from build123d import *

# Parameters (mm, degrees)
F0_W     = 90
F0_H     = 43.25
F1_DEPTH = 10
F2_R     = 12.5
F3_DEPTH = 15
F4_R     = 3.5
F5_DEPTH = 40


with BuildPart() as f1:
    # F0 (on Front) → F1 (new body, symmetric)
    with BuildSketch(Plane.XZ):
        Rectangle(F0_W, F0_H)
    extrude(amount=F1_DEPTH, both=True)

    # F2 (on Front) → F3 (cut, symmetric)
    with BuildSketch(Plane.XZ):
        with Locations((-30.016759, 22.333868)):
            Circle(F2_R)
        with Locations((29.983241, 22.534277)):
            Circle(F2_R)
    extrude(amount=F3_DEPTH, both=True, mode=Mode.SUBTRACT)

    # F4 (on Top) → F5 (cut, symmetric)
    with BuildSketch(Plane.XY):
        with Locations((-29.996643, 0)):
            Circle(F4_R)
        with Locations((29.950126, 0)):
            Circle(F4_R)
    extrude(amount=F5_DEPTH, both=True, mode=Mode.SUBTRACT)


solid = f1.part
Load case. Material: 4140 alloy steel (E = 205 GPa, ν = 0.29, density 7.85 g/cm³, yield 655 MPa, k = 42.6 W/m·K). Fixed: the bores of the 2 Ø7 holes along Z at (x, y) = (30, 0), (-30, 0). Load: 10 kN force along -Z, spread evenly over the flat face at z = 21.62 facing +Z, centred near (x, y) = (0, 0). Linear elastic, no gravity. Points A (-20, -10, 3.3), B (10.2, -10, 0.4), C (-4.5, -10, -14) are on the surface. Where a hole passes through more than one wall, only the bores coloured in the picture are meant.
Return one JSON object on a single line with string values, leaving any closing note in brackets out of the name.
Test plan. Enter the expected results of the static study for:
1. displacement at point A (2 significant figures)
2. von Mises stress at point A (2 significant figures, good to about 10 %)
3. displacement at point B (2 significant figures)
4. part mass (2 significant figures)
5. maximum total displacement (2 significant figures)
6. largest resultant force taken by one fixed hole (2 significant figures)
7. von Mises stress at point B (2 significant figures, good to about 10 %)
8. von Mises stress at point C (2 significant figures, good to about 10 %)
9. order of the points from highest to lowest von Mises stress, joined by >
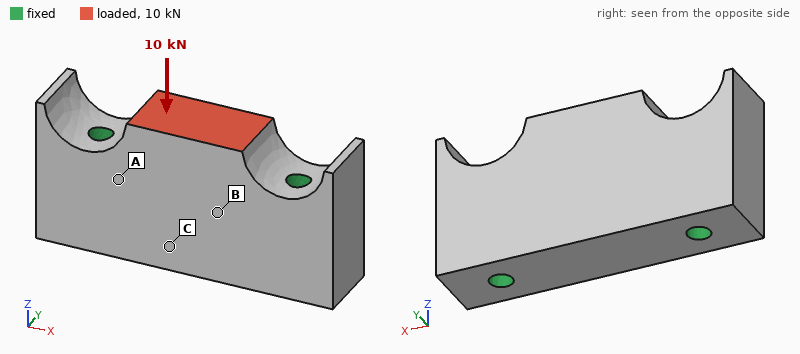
{"displacement at point A": "1.2 µm", "von Mises stress at point A": "15 MPa", "displacement at point B": "1.9 µm", "part mass": "520 g", "maximum total displacement": "3.3 µm", "largest resultant force taken by one fixed hole": "5.3 kN", "von Mises stress at point B": "10 MPa", "von Mises stress at point C": "4.2 MPa", "order of the points from highest to lowest von Mises stress, joined by >": "A > B > C"}
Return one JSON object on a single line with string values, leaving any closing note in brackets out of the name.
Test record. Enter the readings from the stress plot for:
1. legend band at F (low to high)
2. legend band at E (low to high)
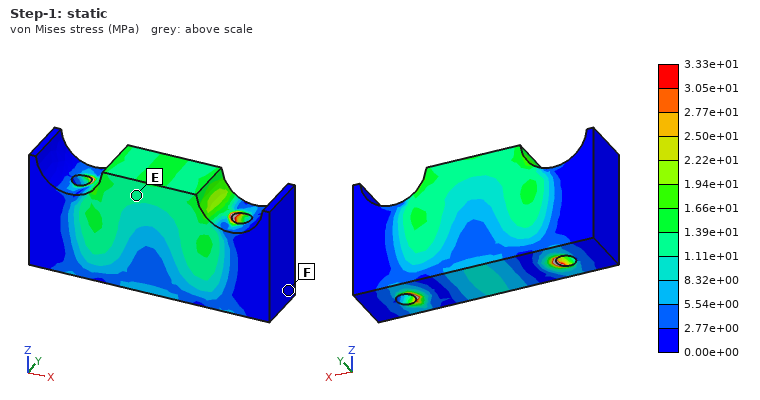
{"legend band at F": "0.00e+00 to 2.77e+00 MPa", "legend band at E": "1.11e+01 to 1.39e+01 MPa"}
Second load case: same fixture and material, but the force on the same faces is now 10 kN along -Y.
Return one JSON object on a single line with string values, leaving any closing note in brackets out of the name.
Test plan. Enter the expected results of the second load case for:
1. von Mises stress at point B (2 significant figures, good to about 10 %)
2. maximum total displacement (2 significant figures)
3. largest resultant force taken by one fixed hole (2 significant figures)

{"von Mises stress at point B": "47 MPa", "maximum total displacement": "24 µm", "largest resultant force taken by one fixed hole": "5.0 kN"}
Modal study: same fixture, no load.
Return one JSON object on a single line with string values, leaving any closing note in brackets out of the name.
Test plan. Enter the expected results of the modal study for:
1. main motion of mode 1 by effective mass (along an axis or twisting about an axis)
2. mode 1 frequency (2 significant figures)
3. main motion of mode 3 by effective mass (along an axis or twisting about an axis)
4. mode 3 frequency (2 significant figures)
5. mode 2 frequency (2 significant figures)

{"main motion of mode 1 by effective mass": "along Y", "mode 1 frequency": "14 kHz", "main motion of mode 3 by effective mass": "along Z", "mode 3 frequency": "22 kHz", "mode 2 frequency": "19 kHz"}
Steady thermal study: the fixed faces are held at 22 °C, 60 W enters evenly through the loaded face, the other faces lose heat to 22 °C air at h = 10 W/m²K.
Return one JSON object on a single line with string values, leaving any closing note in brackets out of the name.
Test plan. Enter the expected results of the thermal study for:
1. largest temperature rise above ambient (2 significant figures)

{"largest temperature rise above ambient": "50 K"}
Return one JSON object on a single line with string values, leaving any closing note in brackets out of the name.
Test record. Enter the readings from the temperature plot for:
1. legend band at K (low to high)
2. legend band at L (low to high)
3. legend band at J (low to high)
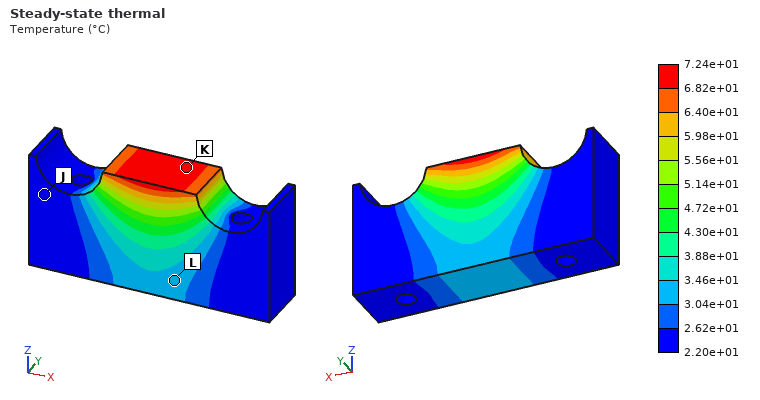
{"legend band at K": "6.82e+01 to 7.24e+01 °C", "legend band at L": "3.04e+01 to 3.46e+01 °C", "legend band at J": "2.20e+01 to 2.62e+01 °C"}
